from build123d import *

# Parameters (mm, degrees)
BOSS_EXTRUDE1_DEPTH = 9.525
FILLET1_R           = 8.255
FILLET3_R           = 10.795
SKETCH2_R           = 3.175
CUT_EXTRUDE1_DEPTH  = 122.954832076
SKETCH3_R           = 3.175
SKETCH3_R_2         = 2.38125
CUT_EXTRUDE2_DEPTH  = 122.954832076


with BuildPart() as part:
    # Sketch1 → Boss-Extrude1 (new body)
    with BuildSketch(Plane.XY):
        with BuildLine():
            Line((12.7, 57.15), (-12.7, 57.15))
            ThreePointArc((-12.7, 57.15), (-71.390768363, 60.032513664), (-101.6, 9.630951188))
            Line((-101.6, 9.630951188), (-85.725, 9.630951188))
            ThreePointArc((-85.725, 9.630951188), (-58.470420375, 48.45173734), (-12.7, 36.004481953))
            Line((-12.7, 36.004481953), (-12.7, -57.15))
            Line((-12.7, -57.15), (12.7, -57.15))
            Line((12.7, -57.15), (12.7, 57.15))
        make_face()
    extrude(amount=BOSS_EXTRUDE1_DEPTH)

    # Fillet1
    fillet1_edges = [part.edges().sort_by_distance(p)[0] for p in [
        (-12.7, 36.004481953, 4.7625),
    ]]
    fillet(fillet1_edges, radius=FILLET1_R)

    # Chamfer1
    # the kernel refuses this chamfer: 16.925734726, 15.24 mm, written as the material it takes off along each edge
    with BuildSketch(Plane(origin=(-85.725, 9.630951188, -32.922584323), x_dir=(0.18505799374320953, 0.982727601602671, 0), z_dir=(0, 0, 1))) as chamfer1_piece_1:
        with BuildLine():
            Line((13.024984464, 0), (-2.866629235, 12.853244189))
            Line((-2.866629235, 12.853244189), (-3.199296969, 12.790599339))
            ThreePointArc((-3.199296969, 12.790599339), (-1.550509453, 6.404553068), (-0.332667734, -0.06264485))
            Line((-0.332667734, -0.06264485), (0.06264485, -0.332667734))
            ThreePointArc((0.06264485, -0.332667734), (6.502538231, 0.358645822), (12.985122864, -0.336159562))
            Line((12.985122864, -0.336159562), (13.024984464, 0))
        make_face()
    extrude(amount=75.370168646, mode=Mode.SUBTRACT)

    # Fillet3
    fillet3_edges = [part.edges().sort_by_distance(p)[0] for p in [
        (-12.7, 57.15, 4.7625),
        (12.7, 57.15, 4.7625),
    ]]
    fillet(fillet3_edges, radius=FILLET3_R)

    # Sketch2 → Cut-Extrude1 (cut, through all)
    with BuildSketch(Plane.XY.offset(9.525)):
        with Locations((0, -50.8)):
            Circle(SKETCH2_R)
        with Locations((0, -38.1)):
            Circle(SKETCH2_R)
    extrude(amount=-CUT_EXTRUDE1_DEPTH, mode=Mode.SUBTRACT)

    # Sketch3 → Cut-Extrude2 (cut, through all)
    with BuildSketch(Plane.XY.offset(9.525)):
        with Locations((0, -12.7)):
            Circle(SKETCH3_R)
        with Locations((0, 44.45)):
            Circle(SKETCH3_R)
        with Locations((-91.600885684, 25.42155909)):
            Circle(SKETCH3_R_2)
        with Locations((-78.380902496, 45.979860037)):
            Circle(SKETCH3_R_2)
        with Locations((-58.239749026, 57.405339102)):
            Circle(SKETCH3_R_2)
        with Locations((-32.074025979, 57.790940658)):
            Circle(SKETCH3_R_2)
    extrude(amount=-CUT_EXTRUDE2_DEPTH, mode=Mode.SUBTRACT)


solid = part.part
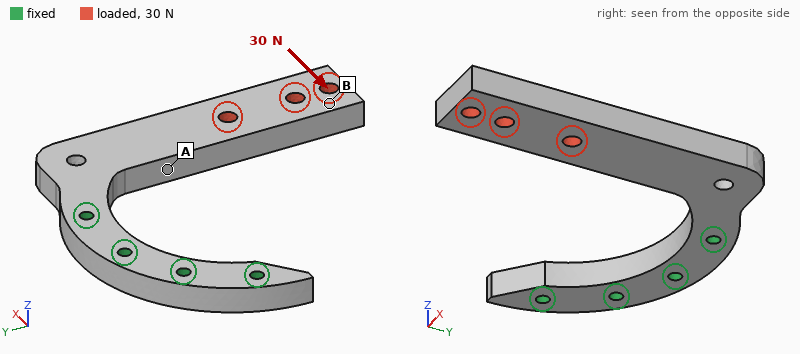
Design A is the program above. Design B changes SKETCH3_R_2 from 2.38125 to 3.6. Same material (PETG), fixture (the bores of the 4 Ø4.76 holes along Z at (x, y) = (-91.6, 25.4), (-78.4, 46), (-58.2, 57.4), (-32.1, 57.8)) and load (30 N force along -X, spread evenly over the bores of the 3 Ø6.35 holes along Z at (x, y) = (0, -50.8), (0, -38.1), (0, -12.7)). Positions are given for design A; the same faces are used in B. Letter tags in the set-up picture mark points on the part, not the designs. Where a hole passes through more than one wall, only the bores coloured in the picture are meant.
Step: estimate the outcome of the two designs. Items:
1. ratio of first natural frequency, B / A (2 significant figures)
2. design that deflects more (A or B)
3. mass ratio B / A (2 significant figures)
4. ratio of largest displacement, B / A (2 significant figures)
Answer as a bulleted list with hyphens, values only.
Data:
- 1.0
- A
- 0.98
- 0.90
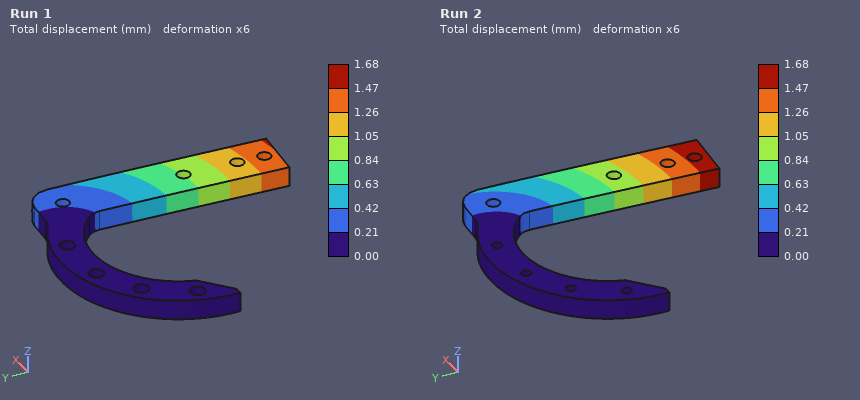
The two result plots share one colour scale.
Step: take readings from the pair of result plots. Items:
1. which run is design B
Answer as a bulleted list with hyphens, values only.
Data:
- Run 1
